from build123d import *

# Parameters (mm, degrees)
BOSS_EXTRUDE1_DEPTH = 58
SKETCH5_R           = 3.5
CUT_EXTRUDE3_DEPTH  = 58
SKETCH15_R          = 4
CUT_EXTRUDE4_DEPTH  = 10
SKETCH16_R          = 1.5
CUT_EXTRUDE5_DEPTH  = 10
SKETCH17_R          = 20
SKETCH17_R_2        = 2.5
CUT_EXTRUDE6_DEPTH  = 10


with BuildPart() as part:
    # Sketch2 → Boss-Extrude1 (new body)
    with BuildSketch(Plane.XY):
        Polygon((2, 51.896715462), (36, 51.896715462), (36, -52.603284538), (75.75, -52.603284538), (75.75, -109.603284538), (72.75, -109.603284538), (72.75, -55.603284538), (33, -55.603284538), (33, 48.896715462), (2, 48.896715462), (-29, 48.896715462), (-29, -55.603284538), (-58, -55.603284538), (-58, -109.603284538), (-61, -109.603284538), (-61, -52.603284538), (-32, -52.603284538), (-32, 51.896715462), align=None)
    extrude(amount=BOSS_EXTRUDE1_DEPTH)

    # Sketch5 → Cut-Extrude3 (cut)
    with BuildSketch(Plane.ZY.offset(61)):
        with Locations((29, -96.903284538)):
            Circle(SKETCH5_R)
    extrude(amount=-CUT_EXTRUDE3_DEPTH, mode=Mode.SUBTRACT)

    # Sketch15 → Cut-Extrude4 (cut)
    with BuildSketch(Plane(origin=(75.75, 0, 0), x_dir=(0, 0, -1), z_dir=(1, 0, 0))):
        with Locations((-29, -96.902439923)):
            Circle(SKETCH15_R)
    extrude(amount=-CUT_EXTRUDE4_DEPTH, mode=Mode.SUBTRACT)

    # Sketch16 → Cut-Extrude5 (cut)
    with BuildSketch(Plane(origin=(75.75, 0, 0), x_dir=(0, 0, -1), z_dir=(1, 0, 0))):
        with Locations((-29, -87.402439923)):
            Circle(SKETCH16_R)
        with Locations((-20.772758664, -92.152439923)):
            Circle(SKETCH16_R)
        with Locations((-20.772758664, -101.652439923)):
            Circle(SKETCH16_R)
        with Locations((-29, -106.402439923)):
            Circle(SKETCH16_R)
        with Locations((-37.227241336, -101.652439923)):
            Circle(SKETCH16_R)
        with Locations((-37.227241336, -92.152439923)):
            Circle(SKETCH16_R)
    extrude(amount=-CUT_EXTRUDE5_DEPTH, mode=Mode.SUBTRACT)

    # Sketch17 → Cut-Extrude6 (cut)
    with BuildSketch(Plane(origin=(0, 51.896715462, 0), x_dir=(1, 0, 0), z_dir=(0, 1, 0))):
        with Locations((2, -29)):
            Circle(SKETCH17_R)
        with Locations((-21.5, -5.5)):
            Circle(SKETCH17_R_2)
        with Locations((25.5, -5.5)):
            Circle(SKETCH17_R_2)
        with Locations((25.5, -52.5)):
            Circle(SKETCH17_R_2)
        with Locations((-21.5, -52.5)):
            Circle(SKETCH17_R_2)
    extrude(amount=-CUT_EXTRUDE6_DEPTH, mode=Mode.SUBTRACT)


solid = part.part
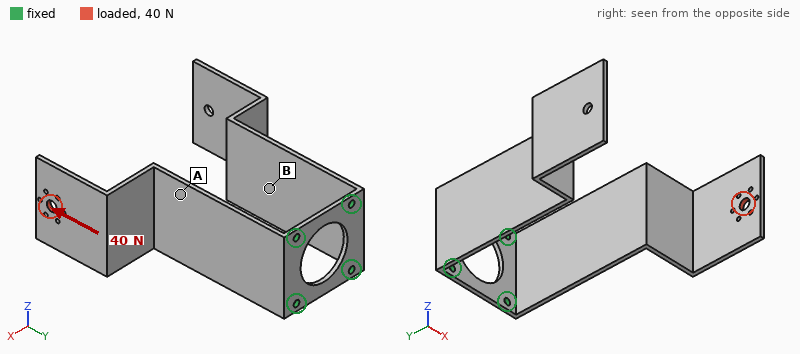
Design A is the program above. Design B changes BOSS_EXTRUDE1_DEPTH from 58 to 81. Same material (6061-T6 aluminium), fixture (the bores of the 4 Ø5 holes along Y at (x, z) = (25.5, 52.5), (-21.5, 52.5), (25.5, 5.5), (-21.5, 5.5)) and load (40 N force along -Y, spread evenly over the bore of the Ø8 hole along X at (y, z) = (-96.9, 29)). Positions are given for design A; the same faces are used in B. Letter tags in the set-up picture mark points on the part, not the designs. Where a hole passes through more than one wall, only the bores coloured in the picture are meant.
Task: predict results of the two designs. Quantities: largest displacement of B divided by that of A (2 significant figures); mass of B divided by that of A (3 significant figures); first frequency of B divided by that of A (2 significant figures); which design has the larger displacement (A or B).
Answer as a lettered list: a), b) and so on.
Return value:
a) 0.72
b) 1.42
c) 1.00
d) A
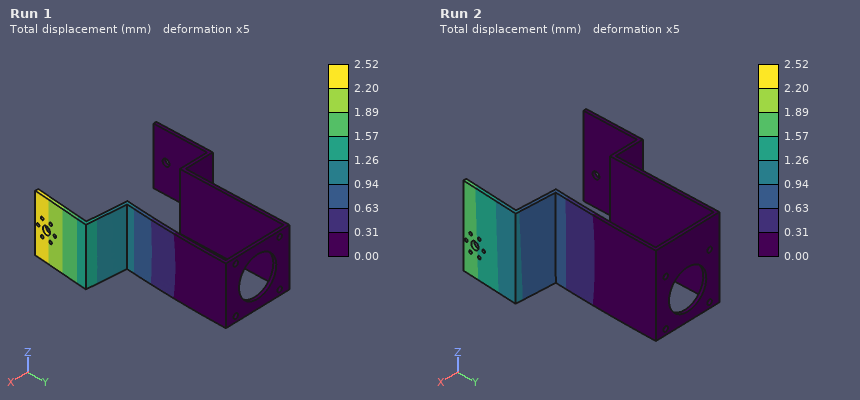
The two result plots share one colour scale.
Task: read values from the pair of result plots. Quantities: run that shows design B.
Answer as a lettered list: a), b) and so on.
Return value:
a) Run 2
